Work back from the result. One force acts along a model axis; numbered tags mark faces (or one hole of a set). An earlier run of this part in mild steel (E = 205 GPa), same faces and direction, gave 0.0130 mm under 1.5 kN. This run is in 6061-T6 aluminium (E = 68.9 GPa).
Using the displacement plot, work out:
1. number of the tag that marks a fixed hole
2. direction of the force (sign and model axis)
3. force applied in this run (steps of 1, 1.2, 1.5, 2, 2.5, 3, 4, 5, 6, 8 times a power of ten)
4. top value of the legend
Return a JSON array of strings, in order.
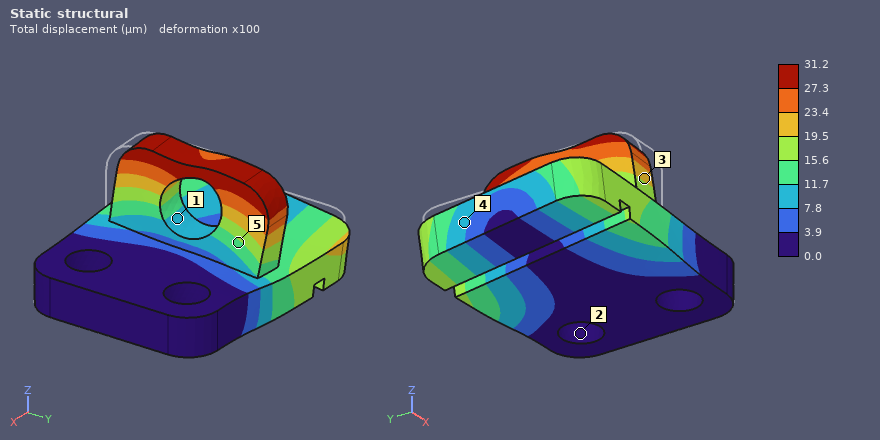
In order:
["2", "+Y", "1.2 kN", "31.2 µm"]
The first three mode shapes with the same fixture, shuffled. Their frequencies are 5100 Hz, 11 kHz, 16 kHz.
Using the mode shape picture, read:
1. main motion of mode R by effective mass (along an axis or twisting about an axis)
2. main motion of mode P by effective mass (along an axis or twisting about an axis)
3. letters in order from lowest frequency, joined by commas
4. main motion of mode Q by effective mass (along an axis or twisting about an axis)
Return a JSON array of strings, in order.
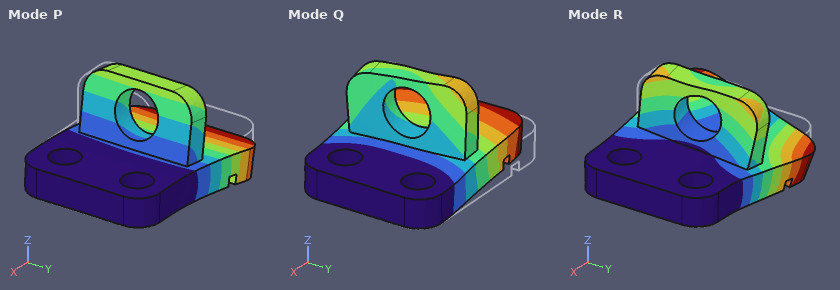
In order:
["twisting about X", "along Z", "P, R, Q", "along Y"]
